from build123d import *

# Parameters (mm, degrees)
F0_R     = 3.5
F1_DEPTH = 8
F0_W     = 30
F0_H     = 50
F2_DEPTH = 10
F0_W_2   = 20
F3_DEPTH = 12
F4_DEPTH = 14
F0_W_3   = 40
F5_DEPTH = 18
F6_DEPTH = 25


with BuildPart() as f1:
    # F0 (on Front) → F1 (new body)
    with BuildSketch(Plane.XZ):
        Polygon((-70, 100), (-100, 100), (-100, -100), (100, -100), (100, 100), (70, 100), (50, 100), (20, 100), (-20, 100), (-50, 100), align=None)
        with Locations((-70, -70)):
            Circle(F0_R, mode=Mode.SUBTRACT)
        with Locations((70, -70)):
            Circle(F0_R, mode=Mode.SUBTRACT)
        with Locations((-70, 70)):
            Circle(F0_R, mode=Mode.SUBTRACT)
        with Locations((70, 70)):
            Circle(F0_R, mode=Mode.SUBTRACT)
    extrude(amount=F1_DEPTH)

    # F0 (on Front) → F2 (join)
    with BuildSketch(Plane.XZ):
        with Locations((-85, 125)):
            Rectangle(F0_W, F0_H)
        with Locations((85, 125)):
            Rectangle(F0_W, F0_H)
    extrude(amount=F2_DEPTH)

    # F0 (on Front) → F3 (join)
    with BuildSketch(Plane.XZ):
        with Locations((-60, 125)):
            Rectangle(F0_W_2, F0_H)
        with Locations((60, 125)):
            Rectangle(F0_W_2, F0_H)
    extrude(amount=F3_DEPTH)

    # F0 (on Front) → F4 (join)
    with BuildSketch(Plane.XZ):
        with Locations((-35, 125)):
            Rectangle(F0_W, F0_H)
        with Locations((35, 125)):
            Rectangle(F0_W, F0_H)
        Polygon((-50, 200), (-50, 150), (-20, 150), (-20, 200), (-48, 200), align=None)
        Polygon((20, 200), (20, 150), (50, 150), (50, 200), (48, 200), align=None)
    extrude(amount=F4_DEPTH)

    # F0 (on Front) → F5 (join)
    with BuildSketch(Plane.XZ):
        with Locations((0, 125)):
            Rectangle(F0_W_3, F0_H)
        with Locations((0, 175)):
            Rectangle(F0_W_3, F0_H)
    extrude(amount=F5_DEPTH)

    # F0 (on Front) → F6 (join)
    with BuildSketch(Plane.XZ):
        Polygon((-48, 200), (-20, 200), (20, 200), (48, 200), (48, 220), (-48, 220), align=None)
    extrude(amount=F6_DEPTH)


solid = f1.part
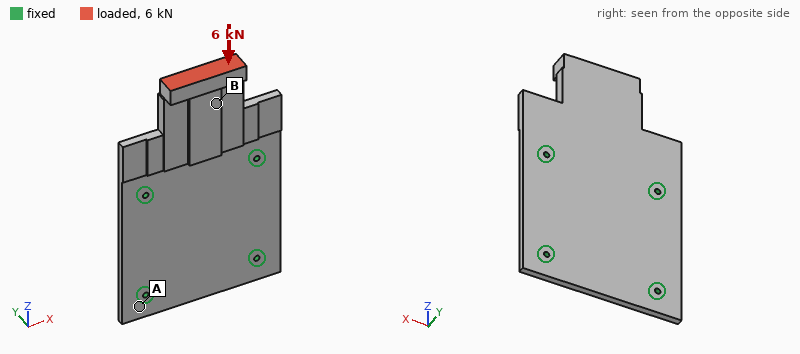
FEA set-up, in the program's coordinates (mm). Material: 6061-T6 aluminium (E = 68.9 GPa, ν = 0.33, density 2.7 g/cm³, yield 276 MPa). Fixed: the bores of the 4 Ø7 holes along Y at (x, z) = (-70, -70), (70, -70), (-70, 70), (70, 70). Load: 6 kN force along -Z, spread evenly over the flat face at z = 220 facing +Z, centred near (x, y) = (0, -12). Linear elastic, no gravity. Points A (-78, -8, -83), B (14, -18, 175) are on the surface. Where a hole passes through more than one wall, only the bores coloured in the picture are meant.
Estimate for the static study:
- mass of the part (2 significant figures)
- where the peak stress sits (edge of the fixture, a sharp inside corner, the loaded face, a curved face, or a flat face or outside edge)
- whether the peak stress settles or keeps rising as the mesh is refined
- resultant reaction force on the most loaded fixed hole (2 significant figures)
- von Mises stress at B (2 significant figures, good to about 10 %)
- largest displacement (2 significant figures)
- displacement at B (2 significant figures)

1.6 kg
edge of the fixture
keeps rising
2.3 kN
12 MPa
0.59 mm
0.37 mm
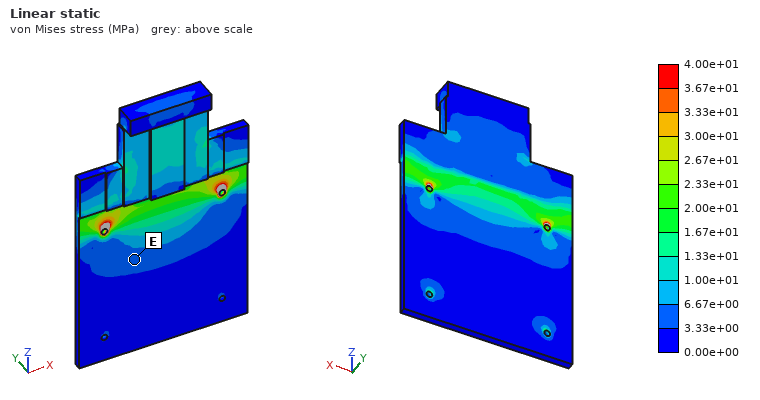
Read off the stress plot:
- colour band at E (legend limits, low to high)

3.33e+00 to 6.67e+00 MPa
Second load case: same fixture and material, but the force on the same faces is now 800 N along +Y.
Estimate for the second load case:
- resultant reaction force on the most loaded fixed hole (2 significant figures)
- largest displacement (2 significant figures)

620 N
1.3 mm
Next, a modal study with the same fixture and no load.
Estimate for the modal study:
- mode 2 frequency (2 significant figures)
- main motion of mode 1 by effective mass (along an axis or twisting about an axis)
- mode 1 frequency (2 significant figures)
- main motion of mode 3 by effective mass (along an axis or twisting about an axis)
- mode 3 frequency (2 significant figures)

1300 Hz
along Y
260 Hz
along Y
1400 Hz
